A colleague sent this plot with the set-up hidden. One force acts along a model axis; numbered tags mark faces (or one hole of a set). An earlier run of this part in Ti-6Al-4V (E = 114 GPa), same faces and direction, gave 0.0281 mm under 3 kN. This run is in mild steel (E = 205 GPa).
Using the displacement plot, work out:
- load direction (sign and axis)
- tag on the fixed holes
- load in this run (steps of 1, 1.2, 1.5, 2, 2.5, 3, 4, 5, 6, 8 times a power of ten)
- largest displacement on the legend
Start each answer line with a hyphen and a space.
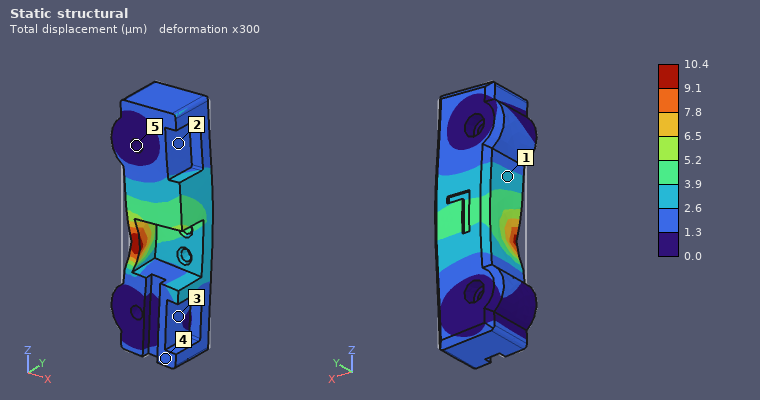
- +X
- 5
- 2 kN
- 10.4 µm
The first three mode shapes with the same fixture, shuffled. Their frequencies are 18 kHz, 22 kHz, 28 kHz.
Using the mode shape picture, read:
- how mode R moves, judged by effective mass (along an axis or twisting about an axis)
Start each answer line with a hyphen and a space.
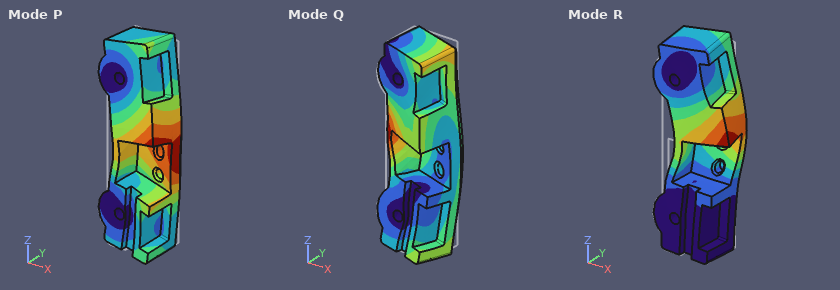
- along Y
